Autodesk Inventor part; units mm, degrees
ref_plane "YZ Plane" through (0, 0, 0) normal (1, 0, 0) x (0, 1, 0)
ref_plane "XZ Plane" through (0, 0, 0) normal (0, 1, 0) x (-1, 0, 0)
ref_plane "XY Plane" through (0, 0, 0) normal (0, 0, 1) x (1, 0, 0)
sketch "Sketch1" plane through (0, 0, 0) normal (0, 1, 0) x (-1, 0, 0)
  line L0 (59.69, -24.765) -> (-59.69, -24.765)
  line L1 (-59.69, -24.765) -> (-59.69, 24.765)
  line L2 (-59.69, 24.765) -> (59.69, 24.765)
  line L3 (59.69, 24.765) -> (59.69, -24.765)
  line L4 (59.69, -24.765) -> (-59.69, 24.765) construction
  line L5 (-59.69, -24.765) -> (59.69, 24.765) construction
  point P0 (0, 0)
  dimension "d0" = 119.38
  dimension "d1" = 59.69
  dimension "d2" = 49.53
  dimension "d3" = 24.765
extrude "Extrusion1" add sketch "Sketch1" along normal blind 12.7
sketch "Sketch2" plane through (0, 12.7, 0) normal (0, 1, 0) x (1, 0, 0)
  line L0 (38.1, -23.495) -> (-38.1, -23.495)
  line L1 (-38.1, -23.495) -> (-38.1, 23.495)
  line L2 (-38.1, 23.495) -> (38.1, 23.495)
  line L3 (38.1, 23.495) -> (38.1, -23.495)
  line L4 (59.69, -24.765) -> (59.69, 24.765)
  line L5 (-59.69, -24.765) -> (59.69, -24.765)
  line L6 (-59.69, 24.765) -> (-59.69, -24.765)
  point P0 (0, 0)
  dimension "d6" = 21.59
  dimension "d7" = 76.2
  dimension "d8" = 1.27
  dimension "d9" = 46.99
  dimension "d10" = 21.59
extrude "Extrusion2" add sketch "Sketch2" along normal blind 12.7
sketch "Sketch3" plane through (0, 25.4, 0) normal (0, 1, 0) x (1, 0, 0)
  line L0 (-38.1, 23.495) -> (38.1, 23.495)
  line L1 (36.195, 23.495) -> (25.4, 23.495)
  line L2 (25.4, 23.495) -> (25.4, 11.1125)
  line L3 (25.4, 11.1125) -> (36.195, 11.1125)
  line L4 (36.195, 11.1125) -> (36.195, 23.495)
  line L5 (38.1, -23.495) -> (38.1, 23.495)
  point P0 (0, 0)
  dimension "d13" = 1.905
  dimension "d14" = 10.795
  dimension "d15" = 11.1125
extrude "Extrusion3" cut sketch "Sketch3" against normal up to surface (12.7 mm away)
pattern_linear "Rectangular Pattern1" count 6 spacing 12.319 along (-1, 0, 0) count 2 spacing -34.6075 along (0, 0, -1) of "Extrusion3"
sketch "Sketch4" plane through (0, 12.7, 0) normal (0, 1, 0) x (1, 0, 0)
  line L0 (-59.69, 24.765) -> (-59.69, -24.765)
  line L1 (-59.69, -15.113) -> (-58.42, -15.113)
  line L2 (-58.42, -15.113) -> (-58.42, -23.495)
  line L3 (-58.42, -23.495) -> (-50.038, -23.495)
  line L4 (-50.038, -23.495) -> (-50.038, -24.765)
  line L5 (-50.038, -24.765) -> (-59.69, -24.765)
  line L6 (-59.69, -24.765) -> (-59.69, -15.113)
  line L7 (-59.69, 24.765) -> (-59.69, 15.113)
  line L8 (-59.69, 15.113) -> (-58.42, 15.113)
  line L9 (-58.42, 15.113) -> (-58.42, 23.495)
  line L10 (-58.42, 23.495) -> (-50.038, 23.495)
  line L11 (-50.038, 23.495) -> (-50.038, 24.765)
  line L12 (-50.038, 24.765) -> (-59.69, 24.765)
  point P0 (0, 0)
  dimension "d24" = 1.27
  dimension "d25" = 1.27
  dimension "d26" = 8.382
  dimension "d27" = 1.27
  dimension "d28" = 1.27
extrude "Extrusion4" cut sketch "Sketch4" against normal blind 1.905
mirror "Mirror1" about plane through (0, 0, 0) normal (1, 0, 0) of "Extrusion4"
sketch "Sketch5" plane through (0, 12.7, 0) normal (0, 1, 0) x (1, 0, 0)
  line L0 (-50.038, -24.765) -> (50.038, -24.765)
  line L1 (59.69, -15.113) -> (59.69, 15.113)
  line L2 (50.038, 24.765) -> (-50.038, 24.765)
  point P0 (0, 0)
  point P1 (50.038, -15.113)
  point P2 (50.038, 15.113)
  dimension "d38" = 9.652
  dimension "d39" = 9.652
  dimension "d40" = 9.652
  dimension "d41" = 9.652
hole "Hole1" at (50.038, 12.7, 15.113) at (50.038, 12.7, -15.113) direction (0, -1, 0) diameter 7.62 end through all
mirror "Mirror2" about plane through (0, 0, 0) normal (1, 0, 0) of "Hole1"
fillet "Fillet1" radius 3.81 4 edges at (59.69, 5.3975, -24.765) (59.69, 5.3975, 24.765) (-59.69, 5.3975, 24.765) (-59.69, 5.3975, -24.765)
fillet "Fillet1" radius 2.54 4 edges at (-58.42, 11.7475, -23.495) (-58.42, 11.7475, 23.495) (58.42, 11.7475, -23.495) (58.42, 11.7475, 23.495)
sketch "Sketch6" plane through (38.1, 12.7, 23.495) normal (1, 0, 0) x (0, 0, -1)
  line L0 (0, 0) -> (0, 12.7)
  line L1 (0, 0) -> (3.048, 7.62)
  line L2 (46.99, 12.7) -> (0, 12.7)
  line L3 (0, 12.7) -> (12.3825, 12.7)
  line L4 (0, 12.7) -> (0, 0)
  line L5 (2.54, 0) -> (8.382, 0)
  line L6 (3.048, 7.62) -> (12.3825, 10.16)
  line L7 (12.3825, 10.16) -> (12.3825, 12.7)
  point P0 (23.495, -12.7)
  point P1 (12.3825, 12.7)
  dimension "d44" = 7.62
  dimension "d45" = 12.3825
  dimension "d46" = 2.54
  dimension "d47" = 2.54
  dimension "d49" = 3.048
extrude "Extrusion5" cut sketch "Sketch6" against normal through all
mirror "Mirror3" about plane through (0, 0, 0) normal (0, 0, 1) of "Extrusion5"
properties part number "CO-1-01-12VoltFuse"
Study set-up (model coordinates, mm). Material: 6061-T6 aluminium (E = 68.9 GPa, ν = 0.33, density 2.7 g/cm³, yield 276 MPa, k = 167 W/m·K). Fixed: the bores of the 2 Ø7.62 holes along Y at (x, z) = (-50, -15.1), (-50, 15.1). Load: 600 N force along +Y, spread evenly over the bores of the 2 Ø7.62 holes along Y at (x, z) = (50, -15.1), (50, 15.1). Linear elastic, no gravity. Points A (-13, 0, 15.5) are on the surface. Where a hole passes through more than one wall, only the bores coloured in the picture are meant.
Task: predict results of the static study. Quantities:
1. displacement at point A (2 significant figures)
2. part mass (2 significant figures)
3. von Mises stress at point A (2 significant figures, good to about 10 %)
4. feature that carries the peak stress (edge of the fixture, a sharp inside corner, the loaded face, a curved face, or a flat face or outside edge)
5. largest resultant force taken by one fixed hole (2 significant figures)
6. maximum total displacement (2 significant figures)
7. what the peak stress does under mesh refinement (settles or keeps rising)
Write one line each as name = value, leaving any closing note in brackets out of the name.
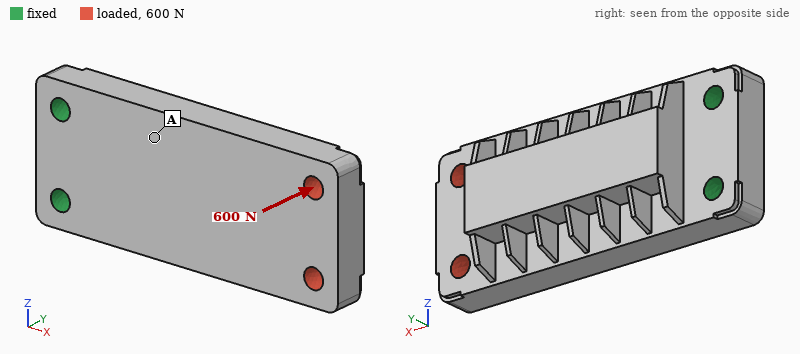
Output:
displacement at point A = 0.053 mm
part mass = 260 g
von Mises stress at point A = 11 MPa
feature that carries the peak stress = edge of the fixture
largest resultant force taken by one fixed hole = 340 N
maximum total displacement = 0.23 mm
what the peak stress does under mesh refinement = keeps rising
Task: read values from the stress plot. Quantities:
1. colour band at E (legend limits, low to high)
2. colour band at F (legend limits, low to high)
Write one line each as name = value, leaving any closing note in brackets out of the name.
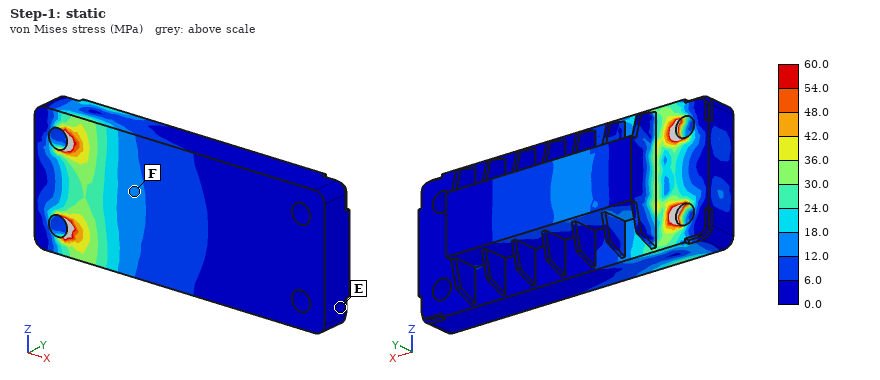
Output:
colour band at E = 0.0 to 6.0 MPa
colour band at F = 12.0 to 18.0 MPa
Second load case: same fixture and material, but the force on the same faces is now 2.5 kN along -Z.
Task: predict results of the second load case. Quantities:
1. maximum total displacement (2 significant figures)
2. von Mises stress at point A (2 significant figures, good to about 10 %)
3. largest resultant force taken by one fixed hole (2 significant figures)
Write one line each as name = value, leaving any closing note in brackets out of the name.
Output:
maximum total displacement = 0.13 mm
von Mises stress at point A = 20 MPa
largest resultant force taken by one fixed hole = 7.4 kN
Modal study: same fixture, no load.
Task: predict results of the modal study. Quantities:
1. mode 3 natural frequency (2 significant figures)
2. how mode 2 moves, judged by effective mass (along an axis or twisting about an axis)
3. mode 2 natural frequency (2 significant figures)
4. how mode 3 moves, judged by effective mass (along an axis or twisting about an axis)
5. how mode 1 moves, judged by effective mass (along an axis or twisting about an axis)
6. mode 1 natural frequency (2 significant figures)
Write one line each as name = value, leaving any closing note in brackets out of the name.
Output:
mode 3 natural frequency = 4600 Hz
how mode 2 moves, judged by effective mass = along Z
mode 2 natural frequency = 2800 Hz
how mode 3 moves, judged by effective mass = twisting about X
how mode 1 moves, judged by effective mass = along Y
mode 1 natural frequency = 980 Hz
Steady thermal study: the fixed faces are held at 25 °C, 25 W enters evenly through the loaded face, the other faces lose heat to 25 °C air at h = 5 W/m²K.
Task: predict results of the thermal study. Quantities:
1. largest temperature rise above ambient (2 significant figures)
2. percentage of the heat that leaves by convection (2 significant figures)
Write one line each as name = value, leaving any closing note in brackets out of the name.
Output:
largest temperature rise above ambient = 20 K
percentage of the heat that leaves by convection = 3.8 %
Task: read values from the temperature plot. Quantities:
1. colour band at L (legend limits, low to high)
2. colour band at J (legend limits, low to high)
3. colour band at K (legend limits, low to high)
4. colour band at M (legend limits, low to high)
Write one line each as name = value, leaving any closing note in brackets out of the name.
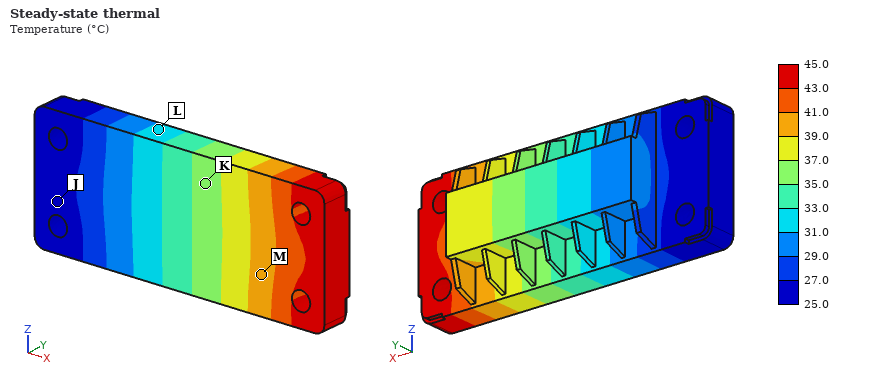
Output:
colour band at L = 31.0 to 33.0 °C
colour band at J = 25.0 to 27.0 °C
colour band at K = 35.0 to 37.0 °C
colour band at M = 39.0 to 41.0 °C
